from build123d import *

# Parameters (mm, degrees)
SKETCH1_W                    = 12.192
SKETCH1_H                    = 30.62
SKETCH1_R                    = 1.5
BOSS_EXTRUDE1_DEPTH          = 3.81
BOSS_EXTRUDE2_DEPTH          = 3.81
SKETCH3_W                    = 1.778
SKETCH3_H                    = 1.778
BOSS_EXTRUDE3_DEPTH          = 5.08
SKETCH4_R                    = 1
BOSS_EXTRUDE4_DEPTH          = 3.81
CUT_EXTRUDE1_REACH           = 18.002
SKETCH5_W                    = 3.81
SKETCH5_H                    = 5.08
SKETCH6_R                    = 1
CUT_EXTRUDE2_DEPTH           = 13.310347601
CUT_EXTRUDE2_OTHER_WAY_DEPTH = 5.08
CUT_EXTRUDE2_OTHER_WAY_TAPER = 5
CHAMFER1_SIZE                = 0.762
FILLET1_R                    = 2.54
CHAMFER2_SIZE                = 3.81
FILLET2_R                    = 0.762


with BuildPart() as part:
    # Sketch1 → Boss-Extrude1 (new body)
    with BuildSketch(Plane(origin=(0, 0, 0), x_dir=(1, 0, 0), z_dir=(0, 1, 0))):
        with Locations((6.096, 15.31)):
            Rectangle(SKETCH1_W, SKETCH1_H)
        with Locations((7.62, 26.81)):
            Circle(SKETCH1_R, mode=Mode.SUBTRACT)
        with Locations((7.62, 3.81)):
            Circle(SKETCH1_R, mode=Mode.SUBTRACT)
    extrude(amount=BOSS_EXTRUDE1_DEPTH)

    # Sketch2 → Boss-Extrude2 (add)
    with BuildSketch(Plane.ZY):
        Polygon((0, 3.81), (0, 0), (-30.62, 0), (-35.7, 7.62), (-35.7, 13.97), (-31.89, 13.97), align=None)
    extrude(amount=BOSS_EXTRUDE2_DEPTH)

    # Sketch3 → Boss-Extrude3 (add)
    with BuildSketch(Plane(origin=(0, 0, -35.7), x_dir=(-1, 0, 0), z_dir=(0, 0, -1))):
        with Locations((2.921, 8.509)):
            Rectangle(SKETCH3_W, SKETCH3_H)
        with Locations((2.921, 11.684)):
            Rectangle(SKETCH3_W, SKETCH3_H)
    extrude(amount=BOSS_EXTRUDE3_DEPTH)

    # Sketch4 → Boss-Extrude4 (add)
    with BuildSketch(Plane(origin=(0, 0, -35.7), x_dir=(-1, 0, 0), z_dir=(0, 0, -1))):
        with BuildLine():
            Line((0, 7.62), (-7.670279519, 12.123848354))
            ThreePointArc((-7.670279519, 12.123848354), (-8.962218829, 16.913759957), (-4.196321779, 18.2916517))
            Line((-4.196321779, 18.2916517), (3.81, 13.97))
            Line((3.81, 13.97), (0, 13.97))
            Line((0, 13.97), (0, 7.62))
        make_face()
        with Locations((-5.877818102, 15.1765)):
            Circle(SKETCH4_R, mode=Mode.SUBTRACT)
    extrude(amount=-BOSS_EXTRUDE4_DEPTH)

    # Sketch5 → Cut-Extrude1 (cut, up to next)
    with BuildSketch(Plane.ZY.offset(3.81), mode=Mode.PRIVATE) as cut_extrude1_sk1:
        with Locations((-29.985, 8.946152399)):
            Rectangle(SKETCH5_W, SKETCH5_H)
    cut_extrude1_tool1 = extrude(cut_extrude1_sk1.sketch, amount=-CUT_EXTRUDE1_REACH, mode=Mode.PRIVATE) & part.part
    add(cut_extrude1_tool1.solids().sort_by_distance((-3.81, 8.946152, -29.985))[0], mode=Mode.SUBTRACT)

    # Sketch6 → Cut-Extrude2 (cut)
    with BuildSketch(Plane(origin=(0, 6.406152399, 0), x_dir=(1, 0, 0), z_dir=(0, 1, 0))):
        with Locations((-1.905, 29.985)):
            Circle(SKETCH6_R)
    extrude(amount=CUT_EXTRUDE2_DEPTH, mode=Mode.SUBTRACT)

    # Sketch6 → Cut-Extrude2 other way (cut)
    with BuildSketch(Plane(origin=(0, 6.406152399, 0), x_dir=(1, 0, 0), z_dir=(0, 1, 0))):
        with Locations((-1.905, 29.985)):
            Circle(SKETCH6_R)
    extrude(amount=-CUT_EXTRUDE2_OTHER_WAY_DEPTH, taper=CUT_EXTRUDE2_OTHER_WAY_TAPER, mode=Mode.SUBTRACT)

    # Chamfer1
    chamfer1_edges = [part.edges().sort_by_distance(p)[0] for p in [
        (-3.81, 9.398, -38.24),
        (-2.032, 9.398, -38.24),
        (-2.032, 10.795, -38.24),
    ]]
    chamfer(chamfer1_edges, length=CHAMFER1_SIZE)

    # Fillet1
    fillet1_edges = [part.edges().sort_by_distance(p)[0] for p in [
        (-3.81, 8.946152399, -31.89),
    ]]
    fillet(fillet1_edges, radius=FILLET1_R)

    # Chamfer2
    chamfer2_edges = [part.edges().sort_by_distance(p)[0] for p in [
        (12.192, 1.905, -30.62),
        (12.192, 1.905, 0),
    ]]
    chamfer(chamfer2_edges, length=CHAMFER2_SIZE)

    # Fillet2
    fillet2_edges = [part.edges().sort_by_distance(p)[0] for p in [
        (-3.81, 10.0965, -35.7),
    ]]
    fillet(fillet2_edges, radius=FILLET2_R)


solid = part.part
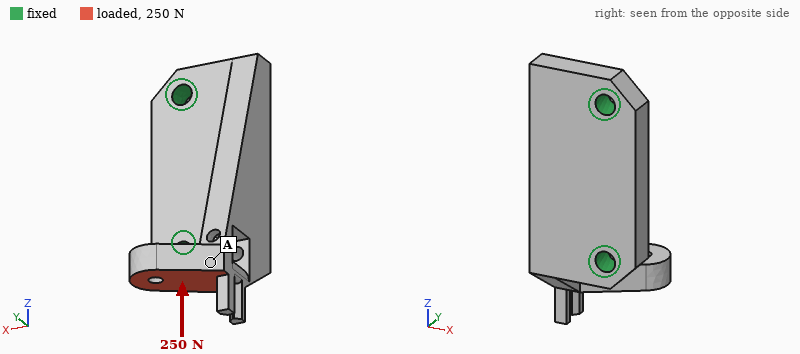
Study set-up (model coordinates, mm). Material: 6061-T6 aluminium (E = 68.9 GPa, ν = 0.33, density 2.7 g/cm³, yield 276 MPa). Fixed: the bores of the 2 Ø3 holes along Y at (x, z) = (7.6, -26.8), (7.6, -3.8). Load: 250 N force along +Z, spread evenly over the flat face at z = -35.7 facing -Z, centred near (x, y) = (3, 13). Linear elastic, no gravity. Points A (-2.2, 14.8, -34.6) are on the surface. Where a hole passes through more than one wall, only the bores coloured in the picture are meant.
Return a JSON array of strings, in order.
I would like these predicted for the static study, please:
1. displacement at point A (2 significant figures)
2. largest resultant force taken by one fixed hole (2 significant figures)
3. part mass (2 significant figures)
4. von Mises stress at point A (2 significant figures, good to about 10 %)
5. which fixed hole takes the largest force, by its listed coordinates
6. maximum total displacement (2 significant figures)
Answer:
["0.055 mm", "210 N", "7.3 g", "25 MPa", "(7.6, -26.8)", "0.14 mm"]
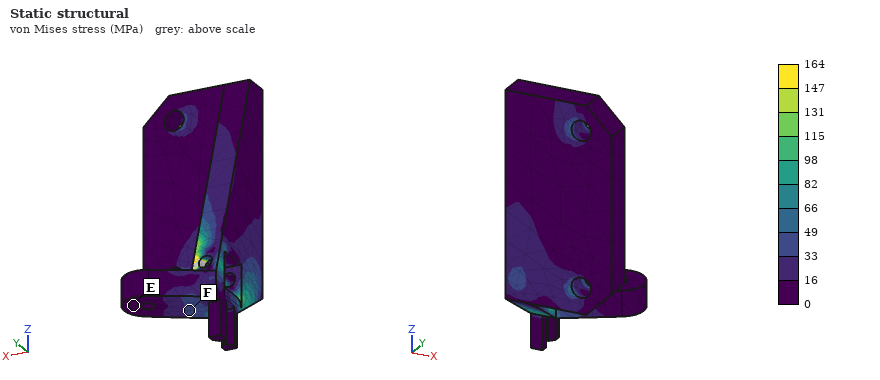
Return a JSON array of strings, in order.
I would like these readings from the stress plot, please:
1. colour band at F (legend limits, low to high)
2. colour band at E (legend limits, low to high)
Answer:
["33 to 49 MPa", "0 to 16 MPa"]
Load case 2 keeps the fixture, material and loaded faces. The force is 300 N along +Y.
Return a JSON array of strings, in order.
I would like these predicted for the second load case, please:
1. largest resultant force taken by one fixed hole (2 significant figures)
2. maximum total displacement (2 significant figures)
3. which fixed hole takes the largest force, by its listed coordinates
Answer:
["410 N", "0.12 mm", "(7.6, -26.8)"]
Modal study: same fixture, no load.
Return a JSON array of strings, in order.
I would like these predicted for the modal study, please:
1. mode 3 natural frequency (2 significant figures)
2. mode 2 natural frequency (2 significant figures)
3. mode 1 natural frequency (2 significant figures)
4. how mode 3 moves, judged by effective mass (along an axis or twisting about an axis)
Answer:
["11 kHz", "9300 Hz", "5600 Hz", "along Y"]
